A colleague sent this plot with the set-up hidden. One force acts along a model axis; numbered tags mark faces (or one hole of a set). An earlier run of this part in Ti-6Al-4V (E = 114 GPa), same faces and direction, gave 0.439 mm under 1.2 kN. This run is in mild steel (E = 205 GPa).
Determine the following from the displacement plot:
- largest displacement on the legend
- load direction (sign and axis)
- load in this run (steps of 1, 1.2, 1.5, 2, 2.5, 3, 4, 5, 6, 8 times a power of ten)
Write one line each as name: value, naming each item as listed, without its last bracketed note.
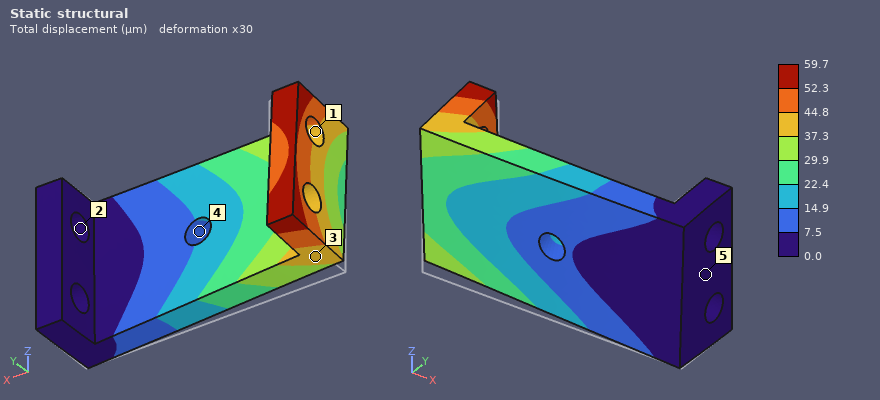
largest displacement on the legend: 59.7 µm
load direction: +Z
load in this run: 300 N
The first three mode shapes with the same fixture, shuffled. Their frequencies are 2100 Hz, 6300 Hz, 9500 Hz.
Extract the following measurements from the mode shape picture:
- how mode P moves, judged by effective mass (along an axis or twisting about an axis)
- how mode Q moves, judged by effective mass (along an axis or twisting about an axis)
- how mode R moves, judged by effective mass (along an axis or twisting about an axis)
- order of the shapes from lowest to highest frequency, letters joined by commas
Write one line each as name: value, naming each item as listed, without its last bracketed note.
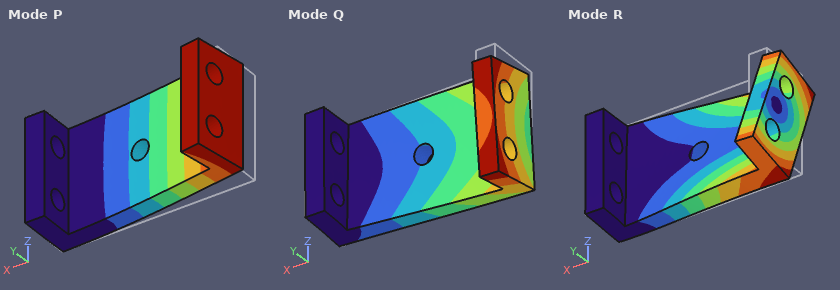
how mode P moves, judged by effective mass: along Y
how mode Q moves, judged by effective mass: along Z
how mode R moves, judged by effective mass: along Z
order of the shapes from lowest to highest frequency, letters joined by commas: P, Q, R
